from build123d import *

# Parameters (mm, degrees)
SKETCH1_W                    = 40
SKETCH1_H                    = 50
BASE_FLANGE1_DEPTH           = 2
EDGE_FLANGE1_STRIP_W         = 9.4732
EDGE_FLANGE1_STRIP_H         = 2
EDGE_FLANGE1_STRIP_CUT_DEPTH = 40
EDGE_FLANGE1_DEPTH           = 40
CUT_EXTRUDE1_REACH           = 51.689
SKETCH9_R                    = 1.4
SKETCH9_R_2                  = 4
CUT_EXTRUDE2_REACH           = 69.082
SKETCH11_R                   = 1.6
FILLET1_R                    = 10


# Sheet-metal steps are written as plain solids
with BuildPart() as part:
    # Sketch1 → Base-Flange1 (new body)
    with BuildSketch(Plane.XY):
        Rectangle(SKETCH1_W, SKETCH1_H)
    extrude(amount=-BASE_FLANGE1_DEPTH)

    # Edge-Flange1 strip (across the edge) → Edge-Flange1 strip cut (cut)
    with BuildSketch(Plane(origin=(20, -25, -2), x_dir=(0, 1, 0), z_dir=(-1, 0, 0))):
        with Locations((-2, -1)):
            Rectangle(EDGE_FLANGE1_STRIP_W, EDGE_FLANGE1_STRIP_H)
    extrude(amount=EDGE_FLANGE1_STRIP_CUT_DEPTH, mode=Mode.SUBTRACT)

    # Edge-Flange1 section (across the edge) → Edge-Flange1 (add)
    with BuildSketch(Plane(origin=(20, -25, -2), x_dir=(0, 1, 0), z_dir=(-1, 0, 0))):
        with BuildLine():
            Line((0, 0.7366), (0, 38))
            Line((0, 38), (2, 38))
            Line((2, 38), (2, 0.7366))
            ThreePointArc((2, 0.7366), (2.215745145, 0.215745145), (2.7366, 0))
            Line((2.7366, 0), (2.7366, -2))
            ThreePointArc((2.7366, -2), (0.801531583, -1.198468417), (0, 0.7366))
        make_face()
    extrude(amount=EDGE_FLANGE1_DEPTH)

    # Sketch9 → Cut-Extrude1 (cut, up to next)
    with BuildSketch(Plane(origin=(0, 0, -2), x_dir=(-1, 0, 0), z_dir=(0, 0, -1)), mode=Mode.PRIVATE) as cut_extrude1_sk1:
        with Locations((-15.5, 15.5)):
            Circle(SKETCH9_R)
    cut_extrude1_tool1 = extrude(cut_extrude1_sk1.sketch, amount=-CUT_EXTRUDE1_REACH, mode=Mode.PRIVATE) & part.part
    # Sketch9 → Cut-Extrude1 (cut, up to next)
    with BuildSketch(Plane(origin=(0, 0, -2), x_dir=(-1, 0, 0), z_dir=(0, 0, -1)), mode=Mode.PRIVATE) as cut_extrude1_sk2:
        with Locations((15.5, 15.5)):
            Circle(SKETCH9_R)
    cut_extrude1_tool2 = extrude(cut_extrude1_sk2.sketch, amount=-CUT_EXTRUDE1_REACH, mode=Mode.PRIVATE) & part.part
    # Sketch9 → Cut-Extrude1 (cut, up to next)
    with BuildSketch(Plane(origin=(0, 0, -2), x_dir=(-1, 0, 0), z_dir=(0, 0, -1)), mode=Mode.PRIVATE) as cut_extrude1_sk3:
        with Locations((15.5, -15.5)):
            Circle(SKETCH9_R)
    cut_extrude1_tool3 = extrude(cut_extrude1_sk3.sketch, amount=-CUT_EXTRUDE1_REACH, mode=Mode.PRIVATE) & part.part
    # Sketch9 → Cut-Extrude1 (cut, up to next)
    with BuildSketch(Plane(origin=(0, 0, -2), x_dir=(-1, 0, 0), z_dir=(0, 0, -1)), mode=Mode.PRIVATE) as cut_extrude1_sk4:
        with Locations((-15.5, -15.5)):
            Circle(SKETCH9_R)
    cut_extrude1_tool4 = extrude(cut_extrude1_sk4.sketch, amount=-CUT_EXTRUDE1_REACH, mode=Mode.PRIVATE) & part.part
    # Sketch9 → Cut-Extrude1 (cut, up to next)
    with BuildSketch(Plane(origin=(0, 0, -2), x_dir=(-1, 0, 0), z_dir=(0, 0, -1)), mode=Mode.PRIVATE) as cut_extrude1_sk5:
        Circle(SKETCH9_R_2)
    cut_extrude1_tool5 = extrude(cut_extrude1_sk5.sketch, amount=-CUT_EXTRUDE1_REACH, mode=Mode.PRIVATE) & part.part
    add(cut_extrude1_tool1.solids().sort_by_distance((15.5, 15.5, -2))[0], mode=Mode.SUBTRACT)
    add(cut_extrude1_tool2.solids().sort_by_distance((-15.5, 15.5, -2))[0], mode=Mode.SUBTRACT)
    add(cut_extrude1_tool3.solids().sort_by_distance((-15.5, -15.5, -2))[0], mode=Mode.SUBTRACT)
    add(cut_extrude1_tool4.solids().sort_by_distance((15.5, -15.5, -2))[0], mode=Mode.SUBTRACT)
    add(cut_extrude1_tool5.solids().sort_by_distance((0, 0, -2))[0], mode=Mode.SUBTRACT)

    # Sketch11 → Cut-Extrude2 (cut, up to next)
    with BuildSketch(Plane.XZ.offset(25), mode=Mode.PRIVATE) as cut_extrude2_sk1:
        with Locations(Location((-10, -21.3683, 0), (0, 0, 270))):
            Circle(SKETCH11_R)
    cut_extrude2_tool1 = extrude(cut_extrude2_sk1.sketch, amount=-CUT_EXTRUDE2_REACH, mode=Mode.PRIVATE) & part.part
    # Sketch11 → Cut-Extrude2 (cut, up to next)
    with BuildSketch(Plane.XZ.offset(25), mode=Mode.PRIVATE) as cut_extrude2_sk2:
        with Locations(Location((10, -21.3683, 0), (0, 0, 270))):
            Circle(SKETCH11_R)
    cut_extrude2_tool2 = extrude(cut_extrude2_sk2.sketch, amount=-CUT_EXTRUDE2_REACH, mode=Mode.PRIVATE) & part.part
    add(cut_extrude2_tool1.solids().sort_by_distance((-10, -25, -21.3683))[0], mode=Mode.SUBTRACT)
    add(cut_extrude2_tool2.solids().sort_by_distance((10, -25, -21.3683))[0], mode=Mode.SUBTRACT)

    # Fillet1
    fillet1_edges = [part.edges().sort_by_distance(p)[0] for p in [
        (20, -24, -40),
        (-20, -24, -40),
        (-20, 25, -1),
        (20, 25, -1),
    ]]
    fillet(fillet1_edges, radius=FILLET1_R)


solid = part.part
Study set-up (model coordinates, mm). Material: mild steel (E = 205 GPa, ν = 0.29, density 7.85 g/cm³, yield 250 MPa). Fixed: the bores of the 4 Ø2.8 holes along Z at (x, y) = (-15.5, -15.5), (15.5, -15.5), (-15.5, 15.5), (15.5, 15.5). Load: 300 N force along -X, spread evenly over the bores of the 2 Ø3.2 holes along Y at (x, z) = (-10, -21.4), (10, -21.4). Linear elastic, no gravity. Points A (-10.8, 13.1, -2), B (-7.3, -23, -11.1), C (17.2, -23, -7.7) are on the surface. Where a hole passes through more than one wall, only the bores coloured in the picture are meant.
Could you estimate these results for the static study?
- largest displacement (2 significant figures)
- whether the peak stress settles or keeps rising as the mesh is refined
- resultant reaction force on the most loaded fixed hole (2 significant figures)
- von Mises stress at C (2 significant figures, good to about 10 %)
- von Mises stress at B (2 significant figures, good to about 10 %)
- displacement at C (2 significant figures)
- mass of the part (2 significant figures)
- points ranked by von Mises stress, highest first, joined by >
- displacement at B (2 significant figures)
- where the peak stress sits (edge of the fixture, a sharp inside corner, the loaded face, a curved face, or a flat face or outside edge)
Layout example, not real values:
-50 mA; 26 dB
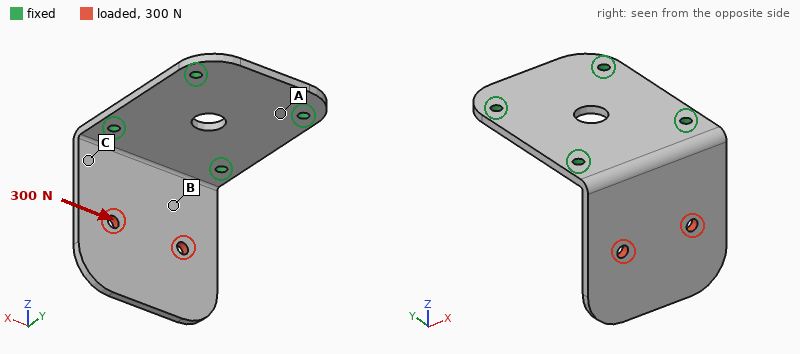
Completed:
43 µm; keeps rising; 260 N; 36 MPa; 22 MPa; 19 µm; 52 g; C > B > A; 13 µm; edge of the fixture
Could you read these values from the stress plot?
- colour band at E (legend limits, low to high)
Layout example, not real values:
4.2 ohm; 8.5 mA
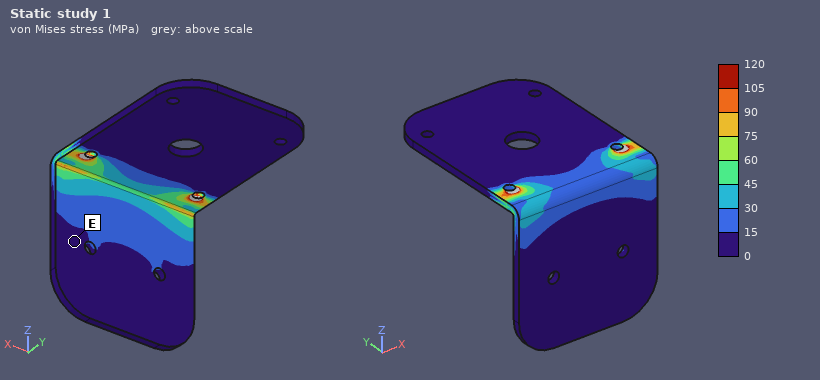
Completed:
0 to 15 MPa
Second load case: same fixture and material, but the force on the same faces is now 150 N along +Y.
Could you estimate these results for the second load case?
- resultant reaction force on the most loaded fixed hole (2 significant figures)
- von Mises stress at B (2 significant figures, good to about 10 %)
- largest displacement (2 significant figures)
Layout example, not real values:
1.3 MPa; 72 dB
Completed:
56 N; 54 MPa; 0.35 mm
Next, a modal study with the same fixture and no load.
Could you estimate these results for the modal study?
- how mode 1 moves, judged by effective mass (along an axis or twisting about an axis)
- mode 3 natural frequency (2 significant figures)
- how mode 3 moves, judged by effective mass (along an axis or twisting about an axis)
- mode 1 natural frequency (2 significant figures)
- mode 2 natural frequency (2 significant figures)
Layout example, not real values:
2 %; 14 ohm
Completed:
along Y; 3900 Hz; along X; 840 Hz; 2400 Hz
